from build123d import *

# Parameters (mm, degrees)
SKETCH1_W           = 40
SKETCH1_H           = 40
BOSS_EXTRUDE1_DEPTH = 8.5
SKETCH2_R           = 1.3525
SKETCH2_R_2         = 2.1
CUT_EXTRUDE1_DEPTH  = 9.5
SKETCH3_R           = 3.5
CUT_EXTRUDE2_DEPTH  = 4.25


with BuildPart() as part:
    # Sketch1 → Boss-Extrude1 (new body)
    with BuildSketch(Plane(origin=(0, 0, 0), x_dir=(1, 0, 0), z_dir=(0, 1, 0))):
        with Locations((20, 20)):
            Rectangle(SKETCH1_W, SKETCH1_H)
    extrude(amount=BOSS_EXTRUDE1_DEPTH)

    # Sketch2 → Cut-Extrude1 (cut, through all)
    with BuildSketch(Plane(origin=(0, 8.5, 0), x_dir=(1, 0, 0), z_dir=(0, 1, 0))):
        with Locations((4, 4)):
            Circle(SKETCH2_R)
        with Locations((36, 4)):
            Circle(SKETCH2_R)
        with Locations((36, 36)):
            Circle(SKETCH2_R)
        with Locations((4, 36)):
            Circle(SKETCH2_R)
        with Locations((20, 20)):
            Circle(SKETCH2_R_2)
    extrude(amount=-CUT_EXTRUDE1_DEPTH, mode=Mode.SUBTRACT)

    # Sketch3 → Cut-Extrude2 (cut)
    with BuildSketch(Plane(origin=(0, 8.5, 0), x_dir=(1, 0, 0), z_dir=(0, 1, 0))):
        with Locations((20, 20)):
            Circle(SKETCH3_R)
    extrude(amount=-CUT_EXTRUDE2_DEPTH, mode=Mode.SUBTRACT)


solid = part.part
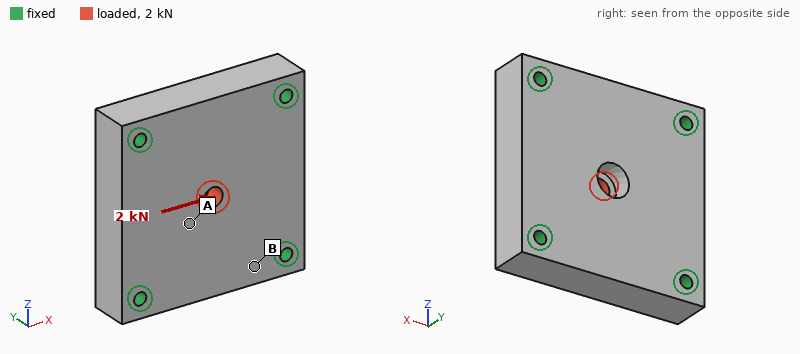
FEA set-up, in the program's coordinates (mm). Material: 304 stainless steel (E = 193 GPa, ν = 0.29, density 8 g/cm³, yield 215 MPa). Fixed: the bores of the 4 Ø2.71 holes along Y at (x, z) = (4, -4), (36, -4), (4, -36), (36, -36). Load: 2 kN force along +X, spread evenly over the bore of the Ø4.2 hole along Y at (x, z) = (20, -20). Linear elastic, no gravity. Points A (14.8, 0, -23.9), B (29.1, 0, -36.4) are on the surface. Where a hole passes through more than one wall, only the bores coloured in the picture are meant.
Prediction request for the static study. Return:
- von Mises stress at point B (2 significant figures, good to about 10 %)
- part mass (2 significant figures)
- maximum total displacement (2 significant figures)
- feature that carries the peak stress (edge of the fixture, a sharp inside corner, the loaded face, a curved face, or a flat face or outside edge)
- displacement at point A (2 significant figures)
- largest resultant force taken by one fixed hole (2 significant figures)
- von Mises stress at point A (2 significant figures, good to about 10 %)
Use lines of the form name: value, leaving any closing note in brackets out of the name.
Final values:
von Mises stress at point B: 4.9 MPa
part mass: 110 g
maximum total displacement: 1.6 µm
feature that carries the peak stress: the loaded face
displacement at point A: 0.92 µm
largest resultant force taken by one fixed hole: 560 N
von Mises stress at point A: 16 MPa
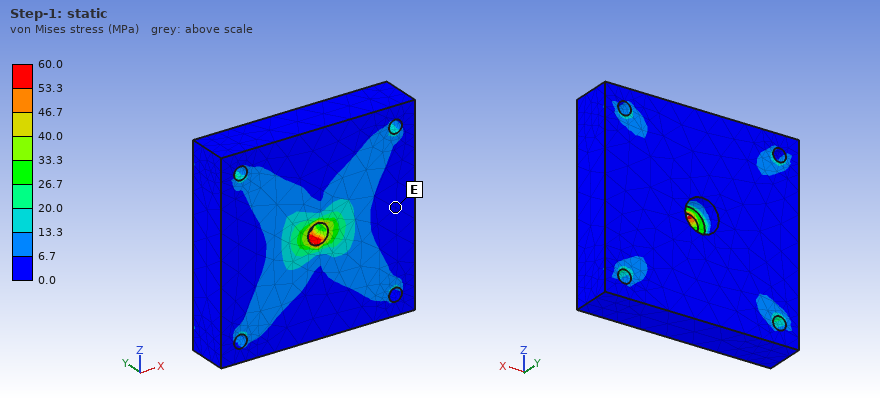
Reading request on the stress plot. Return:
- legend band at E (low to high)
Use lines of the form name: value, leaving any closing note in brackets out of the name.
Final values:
legend band at E: 0.0 to 6.7 MPa
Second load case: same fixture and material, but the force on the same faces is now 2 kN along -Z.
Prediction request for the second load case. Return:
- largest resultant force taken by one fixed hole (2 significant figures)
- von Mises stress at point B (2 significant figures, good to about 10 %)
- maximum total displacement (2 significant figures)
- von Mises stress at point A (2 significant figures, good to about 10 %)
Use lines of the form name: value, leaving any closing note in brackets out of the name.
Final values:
largest resultant force taken by one fixed hole: 560 N
von Mises stress at point B: 4.6 MPa
maximum total displacement: 1.6 µm
von Mises stress at point A: 14 MPa
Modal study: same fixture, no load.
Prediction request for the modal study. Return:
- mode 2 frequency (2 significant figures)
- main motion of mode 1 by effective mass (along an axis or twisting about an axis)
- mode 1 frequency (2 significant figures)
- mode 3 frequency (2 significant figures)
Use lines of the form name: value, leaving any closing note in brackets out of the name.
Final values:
mode 2 frequency: 31 kHz
main motion of mode 1 by effective mass: along Y
mode 1 frequency: 20 kHz
mode 3 frequency: 31 kHz
